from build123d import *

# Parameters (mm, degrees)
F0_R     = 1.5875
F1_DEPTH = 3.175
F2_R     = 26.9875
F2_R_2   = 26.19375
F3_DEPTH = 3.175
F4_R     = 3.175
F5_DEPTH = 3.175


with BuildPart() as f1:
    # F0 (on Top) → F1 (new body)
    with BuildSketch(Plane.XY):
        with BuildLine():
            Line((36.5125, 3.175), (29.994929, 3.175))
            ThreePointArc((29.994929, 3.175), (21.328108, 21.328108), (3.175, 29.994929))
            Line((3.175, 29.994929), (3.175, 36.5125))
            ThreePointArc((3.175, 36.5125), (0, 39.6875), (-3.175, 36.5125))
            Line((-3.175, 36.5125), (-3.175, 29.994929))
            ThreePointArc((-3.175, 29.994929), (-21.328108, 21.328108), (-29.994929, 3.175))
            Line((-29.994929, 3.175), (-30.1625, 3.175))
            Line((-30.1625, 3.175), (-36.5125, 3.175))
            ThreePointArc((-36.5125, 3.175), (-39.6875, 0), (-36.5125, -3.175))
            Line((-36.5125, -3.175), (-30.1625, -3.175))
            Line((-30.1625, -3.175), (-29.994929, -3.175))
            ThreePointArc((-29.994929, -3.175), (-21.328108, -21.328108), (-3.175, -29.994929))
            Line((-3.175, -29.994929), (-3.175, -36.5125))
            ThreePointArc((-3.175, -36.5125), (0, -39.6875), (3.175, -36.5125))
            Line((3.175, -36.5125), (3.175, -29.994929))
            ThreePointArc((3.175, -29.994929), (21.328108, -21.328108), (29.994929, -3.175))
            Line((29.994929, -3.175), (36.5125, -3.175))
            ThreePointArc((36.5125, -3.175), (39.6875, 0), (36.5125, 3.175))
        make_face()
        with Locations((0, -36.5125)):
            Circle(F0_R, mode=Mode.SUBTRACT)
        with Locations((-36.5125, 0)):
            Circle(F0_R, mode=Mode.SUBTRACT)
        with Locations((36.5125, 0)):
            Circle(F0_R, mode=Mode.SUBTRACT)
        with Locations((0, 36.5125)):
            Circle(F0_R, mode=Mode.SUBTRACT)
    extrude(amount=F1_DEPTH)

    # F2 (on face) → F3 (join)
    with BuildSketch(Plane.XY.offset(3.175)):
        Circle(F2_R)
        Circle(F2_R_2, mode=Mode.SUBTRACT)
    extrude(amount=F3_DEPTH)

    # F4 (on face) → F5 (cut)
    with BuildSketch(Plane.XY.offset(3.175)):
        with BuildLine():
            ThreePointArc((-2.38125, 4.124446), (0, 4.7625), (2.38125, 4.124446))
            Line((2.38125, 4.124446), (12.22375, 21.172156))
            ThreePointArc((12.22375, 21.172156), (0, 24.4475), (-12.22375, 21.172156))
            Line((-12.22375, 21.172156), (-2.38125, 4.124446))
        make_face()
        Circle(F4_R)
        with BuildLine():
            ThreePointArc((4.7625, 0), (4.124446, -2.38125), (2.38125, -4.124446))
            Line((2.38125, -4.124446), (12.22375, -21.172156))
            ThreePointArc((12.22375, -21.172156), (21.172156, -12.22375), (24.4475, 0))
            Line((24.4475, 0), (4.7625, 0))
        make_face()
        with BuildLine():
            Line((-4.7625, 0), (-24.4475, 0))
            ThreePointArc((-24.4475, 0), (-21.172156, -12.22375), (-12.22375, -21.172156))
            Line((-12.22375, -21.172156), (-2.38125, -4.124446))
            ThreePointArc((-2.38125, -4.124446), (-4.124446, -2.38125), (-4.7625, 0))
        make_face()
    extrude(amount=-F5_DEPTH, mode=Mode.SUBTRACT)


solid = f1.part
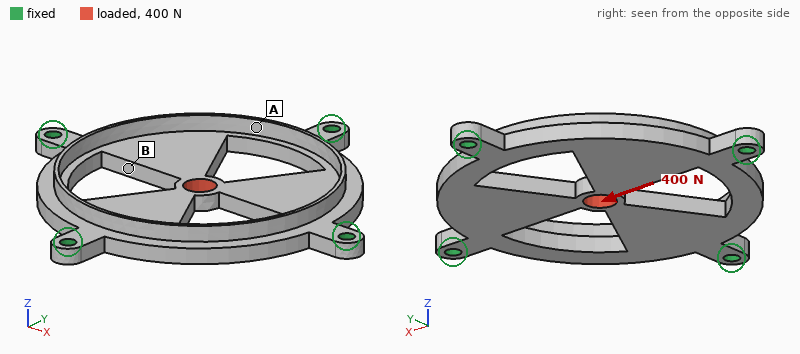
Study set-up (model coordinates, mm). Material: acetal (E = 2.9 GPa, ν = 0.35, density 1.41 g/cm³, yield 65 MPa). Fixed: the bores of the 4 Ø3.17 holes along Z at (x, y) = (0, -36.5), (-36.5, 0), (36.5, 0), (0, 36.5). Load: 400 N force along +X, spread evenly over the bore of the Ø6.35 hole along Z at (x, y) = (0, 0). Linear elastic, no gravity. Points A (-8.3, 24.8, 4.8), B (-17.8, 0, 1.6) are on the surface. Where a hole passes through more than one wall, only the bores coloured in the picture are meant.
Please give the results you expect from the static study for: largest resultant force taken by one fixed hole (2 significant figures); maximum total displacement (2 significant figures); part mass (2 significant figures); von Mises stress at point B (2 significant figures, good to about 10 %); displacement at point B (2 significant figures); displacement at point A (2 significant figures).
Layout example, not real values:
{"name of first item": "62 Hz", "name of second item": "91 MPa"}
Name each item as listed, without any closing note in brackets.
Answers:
{"largest resultant force taken by one fixed hole": "150 N", "maximum total displacement": "0.26 mm", "part mass": "10 g", "von Mises stress at point B": "12 MPa", "displacement at point B": "0.080 mm", "displacement at point A": "0.068 mm"}
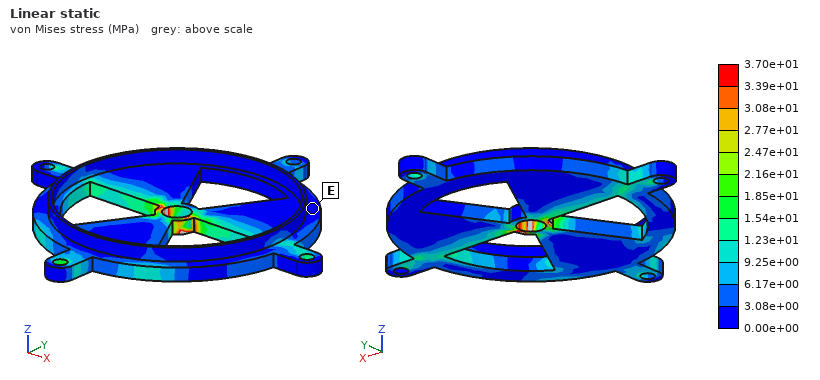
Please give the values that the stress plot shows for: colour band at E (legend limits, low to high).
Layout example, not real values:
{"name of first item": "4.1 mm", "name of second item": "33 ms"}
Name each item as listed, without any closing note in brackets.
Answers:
{"colour band at E": "0.00e+00 to 3.08e+00 MPa"}
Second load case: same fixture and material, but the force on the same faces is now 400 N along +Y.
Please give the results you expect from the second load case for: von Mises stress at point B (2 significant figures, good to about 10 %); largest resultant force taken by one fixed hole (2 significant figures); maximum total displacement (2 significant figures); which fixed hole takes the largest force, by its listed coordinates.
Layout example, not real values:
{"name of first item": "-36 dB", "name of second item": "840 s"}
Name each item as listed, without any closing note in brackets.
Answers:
{"von Mises stress at point B": "3.2 MPa", "largest resultant force taken by one fixed hole": "250 N", "maximum total displacement": "0.23 mm", "which fixed hole takes the largest force, by its listed coordinates": "(0, -36.5)"}
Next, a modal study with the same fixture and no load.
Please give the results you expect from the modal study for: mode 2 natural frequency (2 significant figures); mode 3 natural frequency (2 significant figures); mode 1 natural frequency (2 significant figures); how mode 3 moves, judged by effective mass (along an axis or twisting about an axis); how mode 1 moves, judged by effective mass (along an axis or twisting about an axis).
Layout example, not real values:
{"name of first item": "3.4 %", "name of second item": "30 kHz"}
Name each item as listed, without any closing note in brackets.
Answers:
{"mode 2 natural frequency": "1500 Hz", "mode 3 natural frequency": "1700 Hz", "mode 1 natural frequency": "1000 Hz", "how mode 3 moves, judged by effective mass": "twisting about X", "how mode 1 moves, judged by effective mass": "along Z"}
